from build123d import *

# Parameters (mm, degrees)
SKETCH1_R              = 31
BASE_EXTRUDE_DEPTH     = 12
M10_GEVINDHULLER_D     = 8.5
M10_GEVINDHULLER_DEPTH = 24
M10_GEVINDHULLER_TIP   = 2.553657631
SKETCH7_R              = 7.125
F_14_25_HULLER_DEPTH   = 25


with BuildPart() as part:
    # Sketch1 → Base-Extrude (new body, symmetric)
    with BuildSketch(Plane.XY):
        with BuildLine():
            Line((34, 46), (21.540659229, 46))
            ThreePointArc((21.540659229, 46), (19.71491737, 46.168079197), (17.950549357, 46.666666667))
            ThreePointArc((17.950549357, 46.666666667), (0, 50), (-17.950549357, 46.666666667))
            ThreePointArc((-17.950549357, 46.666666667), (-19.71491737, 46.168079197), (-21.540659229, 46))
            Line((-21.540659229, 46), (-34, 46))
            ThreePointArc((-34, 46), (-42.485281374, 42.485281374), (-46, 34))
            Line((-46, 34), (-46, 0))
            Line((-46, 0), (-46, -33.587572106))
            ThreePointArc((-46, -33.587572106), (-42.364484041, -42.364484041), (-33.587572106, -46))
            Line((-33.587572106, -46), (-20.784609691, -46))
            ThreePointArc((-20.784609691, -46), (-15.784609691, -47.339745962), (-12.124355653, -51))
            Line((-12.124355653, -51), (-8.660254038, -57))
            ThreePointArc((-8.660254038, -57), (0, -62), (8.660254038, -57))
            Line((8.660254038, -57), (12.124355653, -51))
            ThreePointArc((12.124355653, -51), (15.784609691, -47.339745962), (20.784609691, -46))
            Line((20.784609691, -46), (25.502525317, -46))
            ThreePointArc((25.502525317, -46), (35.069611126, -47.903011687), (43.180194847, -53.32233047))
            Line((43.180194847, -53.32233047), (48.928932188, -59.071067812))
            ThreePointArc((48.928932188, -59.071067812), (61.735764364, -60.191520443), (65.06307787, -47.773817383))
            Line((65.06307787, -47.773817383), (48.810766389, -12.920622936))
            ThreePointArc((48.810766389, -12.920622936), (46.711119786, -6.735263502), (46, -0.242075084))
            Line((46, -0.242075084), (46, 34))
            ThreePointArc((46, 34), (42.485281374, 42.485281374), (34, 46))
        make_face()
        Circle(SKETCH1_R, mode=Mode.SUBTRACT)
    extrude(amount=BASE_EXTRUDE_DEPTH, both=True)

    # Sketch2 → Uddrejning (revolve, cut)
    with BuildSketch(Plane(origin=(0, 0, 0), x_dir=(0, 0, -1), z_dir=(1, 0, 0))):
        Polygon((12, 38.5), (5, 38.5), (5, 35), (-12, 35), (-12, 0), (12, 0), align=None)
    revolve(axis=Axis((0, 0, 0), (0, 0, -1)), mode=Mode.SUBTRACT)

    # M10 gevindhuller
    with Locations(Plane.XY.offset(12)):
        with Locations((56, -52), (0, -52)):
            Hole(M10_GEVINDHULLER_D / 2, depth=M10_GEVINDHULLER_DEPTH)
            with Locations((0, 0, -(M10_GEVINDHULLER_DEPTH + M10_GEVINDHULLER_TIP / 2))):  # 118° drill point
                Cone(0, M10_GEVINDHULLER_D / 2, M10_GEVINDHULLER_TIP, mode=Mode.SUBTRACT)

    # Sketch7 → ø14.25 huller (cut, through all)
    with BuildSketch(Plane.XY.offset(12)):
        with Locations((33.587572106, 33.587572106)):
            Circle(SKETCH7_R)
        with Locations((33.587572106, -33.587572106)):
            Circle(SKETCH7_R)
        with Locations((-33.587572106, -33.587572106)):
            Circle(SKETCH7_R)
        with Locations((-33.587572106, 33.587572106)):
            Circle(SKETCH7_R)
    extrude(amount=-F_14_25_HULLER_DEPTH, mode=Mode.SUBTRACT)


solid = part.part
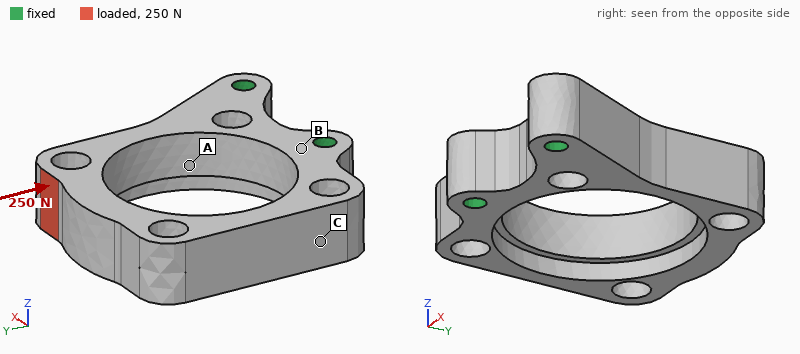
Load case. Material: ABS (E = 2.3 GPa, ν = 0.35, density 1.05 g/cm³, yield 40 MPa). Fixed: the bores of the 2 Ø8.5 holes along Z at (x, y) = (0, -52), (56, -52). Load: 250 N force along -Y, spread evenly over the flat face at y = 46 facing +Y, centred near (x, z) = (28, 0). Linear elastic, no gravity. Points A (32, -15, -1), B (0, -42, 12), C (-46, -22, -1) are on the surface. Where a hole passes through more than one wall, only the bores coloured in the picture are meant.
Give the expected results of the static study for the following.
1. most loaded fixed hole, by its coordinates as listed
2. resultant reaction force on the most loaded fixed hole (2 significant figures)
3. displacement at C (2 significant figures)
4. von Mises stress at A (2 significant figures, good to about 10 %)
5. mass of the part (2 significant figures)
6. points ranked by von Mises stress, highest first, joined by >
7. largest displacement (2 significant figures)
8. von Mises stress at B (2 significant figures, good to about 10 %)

(56, -52)
150 N
0.10 mm
1.1 MPa
120 g
A > B > C
0.16 mm
0.54 MPa
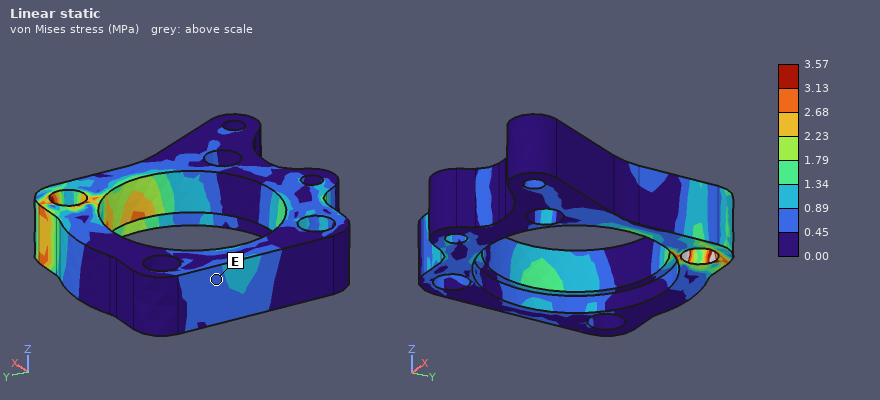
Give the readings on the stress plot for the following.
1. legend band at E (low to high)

0.45 to 0.89 MPa
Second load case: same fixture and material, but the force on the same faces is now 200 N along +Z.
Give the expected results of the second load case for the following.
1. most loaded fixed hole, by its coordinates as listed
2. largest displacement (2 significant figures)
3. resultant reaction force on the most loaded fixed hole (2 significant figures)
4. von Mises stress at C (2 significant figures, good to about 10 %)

(56, -52)
1.2 mm
130 N
0.85 MPa
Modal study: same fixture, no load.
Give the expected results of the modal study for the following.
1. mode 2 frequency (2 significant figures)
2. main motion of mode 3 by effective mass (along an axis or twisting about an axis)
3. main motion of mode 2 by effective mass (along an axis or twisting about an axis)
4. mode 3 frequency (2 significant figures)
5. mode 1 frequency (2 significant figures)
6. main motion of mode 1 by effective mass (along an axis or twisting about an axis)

480 Hz
twisting about Y
along X
780 Hz
350 Hz
along Z
